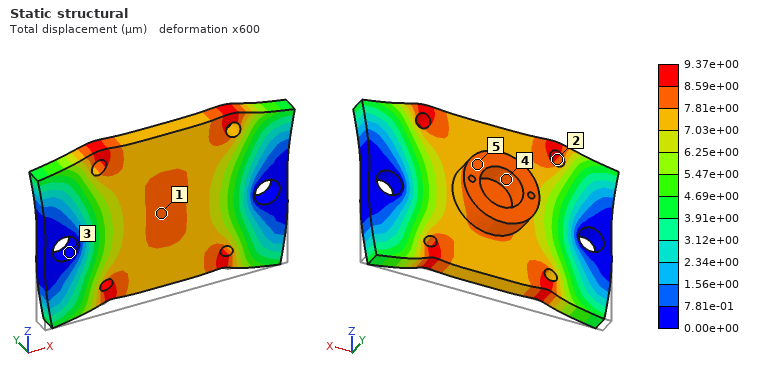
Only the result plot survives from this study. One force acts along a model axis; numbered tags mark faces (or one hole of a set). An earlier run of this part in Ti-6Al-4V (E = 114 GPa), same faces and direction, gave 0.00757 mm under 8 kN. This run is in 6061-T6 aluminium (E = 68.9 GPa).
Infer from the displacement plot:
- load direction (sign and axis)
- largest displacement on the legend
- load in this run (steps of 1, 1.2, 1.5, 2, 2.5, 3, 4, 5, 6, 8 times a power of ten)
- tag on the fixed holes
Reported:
+Z
9.37e+00 µm
6 kN
3
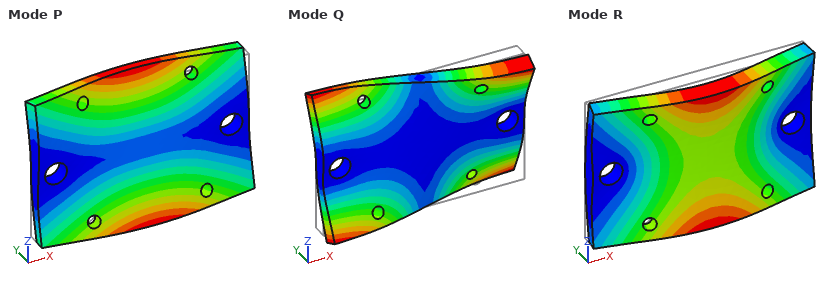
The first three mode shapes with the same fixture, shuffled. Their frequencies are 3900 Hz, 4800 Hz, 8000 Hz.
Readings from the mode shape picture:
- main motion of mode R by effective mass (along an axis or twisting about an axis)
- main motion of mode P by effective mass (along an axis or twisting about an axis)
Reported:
along Y
twisting about X
